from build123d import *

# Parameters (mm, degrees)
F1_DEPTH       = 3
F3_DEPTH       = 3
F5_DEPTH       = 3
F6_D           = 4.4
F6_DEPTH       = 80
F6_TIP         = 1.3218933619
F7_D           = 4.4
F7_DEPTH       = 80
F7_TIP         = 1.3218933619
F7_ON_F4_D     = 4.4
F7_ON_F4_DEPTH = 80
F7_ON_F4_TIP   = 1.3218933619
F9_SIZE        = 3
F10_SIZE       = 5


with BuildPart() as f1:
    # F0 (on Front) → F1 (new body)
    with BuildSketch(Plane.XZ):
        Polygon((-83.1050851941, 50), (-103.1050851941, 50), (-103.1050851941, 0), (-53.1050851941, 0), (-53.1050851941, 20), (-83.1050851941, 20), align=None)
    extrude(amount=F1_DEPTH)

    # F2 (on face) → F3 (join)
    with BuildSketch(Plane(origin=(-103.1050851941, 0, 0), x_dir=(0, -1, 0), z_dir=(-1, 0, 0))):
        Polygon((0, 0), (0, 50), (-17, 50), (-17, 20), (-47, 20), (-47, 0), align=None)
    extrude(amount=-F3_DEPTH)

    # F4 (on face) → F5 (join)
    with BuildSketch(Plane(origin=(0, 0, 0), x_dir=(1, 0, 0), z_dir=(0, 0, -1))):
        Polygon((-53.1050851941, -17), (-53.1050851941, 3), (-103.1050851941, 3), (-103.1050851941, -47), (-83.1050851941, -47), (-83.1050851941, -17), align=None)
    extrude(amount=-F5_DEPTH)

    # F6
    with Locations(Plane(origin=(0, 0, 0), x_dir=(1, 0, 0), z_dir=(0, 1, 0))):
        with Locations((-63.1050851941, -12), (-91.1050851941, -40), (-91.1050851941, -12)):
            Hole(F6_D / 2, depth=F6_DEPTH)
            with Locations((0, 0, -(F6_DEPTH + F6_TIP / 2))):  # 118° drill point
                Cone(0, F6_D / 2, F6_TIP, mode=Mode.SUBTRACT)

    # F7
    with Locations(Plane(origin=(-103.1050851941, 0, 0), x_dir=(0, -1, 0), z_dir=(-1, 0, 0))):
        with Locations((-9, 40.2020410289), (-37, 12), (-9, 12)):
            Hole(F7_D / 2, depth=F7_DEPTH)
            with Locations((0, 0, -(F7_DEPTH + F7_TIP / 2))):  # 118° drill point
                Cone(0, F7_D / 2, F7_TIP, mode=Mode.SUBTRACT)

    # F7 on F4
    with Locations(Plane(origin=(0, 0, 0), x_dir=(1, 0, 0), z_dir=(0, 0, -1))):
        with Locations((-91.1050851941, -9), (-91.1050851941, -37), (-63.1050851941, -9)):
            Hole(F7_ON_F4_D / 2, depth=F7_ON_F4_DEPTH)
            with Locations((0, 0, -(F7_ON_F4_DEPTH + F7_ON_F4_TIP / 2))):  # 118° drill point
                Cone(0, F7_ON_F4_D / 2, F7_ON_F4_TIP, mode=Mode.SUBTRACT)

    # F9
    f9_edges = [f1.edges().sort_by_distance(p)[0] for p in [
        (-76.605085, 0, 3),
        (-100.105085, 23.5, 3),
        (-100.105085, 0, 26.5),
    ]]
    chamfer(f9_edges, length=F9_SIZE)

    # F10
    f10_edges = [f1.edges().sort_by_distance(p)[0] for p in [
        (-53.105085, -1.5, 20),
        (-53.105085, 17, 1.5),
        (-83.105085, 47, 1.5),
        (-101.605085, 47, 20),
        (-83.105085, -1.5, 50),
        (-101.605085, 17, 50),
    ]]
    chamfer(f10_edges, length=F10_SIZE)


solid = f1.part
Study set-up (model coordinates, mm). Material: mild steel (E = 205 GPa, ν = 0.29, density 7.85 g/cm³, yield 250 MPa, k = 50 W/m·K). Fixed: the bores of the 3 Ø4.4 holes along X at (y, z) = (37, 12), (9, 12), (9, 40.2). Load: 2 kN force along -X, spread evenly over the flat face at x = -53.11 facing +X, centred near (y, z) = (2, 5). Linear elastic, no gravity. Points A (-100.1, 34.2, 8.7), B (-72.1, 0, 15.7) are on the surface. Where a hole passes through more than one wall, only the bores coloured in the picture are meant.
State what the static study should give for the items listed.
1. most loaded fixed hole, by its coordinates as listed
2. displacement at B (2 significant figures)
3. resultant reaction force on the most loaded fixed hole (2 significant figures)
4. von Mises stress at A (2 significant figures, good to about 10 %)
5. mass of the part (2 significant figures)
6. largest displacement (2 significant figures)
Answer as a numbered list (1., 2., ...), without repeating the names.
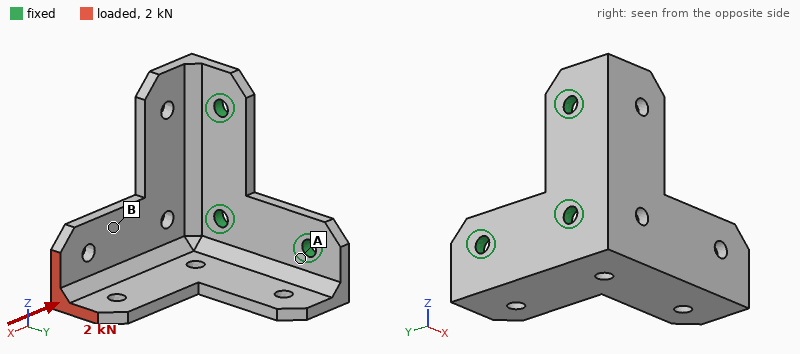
1. (9, 12)
2. 42 µm
3. 2.6 kN
4. 42 MPa
5. 100 g
6. 77 µm
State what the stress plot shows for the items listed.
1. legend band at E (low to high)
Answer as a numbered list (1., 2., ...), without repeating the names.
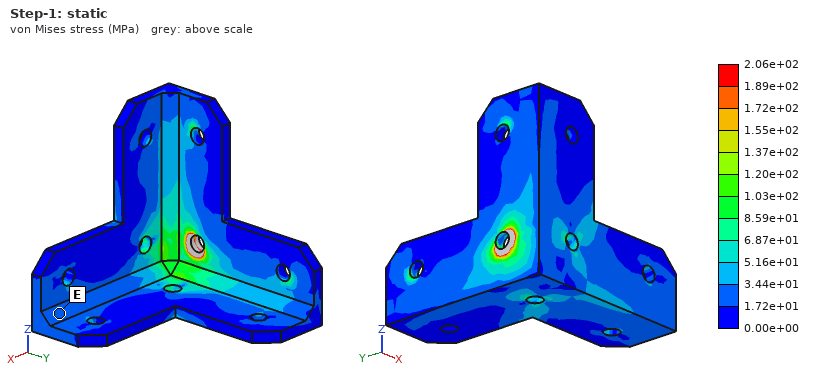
1. 1.72e+01 to 3.44e+01 MPa
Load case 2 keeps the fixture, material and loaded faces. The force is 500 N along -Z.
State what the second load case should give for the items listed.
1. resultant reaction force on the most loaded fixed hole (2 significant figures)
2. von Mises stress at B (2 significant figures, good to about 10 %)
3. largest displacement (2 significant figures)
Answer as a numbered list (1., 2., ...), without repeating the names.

1. 900 N
2. 35 MPa
3. 0.10 mm
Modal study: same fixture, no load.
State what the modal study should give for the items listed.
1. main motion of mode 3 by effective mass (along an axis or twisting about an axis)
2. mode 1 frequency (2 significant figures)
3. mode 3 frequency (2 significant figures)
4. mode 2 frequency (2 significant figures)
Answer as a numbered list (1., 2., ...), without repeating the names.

1. along X
2. 3200 Hz
3. 6400 Hz
4. 3200 Hz
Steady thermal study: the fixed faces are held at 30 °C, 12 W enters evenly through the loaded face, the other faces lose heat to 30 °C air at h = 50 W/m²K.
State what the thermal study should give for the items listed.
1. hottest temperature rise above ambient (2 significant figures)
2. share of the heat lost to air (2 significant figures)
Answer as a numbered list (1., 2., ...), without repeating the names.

1. 77 K
2. 57 %
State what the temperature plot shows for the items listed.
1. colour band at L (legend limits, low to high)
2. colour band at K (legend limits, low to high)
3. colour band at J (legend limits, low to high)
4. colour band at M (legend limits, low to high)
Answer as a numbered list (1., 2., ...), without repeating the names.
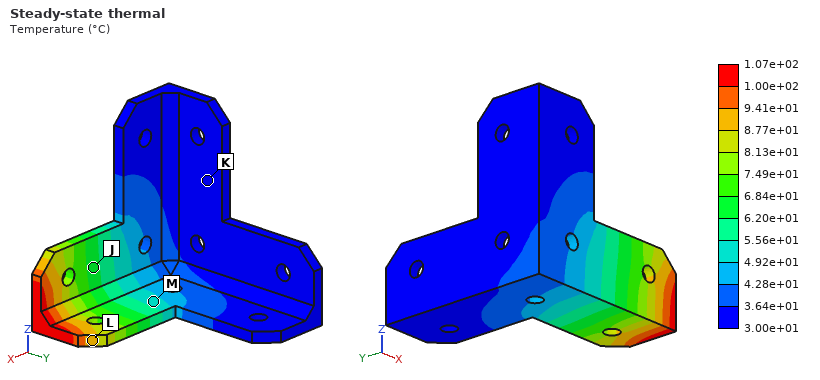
1. 8.77e+01 to 9.41e+01 °C
2. 3.00e+01 to 3.64e+01 °C
3. 6.20e+01 to 6.84e+01 °C
4. 4.92e+01 to 5.56e+01 °C
